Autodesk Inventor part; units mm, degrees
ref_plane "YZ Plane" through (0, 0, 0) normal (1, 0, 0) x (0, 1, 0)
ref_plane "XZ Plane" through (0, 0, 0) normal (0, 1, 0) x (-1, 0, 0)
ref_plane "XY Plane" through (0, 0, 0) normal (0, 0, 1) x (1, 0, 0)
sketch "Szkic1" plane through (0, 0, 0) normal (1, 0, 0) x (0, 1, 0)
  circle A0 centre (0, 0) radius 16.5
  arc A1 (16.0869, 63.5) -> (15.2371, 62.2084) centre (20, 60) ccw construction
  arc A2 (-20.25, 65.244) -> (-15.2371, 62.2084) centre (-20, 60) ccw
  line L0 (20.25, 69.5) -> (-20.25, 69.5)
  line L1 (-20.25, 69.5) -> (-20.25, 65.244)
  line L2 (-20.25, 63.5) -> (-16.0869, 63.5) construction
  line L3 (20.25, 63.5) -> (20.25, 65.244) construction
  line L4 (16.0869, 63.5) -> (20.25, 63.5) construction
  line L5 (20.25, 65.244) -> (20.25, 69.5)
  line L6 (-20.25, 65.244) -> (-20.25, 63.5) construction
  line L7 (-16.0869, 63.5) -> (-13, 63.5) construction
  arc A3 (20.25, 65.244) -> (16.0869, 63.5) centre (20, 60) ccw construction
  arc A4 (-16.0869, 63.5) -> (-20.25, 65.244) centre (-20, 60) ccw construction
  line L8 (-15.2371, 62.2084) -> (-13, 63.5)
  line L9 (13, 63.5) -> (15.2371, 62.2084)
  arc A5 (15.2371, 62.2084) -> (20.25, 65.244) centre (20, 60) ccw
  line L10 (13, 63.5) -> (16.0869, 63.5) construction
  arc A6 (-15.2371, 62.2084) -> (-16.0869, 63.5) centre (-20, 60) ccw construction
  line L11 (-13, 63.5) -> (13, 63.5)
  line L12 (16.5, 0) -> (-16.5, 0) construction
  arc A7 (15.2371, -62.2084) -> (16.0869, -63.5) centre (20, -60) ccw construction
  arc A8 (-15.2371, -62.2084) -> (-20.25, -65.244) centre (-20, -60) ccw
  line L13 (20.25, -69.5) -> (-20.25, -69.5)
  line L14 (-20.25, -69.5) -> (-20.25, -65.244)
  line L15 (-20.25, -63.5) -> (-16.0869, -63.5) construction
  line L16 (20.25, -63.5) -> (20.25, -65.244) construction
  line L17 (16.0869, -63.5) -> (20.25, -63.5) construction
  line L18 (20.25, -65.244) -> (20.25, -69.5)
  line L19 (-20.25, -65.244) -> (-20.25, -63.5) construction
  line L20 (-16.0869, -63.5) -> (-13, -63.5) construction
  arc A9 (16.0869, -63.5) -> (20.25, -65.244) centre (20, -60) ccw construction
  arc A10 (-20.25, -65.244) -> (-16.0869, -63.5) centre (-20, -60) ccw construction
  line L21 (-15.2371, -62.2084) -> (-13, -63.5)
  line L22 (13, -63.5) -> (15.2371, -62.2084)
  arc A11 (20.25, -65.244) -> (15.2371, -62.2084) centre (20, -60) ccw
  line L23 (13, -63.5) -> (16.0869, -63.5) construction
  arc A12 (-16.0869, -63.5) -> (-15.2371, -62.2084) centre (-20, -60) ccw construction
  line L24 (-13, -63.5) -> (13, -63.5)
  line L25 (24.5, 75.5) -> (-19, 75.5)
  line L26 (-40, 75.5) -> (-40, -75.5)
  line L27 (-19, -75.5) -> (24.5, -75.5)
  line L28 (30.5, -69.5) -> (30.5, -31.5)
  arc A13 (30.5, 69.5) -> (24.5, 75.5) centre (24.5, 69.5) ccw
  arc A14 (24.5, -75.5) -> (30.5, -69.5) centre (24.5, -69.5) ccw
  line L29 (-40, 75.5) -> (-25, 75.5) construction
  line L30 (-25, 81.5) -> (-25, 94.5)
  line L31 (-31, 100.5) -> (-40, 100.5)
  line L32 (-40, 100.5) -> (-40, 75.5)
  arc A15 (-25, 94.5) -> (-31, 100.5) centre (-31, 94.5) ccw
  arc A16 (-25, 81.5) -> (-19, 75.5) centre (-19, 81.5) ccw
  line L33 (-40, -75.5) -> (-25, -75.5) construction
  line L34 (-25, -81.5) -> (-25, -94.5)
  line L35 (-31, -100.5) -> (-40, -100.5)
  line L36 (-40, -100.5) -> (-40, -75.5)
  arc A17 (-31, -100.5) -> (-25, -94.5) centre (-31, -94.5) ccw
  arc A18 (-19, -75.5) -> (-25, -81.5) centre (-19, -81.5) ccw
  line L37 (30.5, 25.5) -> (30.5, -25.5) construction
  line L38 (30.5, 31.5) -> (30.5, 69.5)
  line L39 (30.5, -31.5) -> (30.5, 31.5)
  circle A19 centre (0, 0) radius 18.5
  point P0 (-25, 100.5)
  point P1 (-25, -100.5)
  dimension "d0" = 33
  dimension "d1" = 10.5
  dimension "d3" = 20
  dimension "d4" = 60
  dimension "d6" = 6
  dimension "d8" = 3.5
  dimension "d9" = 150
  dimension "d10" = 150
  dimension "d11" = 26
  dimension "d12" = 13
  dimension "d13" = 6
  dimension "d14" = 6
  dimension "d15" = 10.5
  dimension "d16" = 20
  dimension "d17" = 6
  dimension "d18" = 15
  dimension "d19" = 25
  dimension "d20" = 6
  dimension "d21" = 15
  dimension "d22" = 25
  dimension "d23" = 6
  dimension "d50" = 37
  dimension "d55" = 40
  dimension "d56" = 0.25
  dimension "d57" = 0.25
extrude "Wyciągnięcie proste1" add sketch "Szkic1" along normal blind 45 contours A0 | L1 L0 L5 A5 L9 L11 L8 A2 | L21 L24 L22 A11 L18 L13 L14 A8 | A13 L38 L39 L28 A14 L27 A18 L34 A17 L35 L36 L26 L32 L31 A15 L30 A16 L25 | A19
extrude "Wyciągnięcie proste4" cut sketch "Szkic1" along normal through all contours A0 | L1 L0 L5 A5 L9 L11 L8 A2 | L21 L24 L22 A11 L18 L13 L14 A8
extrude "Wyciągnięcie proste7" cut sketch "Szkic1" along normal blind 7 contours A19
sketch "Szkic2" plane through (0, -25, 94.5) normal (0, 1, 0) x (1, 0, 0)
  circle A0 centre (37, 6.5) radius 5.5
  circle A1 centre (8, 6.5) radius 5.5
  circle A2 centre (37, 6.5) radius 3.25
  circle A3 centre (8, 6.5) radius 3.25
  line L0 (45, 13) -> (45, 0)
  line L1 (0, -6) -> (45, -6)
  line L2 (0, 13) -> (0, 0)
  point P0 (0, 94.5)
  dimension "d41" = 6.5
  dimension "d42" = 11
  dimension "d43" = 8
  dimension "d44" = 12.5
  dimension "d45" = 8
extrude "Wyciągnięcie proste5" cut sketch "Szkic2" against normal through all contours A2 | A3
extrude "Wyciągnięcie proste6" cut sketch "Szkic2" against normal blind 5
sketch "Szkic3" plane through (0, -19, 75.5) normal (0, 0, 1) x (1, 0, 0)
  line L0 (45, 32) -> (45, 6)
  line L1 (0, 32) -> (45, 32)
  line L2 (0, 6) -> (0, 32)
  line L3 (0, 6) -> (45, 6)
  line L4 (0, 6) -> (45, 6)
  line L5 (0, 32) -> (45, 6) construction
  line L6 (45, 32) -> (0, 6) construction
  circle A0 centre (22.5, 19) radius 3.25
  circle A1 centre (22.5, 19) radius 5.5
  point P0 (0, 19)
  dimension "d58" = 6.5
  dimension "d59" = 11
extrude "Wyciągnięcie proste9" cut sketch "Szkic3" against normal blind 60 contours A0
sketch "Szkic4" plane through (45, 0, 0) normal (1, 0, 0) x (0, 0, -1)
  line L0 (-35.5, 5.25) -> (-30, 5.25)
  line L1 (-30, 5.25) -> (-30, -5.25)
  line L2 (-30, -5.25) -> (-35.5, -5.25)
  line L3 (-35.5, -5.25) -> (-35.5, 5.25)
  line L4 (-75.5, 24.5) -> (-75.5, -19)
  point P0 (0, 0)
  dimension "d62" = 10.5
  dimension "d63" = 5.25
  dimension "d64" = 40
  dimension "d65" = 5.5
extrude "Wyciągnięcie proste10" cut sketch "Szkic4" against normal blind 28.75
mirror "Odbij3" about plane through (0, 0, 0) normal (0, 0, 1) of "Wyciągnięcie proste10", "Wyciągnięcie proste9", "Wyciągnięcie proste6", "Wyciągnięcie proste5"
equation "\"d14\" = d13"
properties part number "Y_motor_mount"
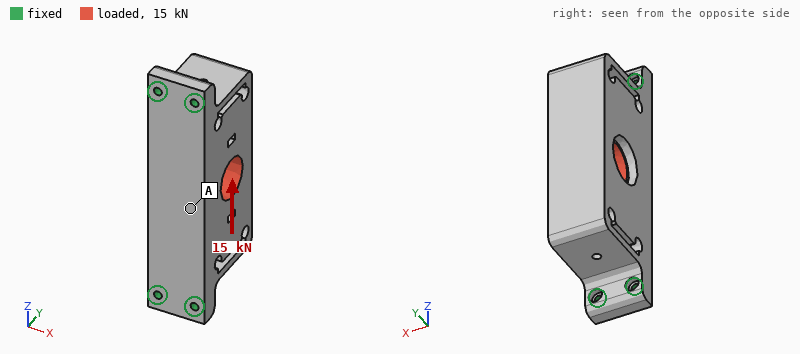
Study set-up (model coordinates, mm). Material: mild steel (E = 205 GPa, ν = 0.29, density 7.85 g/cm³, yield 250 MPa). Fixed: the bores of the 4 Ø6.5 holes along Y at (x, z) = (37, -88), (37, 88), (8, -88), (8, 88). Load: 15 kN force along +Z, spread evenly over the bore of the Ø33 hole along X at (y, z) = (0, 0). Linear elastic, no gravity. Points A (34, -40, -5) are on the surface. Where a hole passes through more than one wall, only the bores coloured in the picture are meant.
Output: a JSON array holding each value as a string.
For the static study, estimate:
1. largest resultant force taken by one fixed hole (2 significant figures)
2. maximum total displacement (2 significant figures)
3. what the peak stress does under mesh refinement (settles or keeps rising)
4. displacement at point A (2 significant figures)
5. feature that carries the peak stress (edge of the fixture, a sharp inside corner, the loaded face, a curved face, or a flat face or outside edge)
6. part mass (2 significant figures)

["4.3 kN", "10 µm", "keeps rising", "2.2 µm", "edge of the fixture", "3.3 kg"]
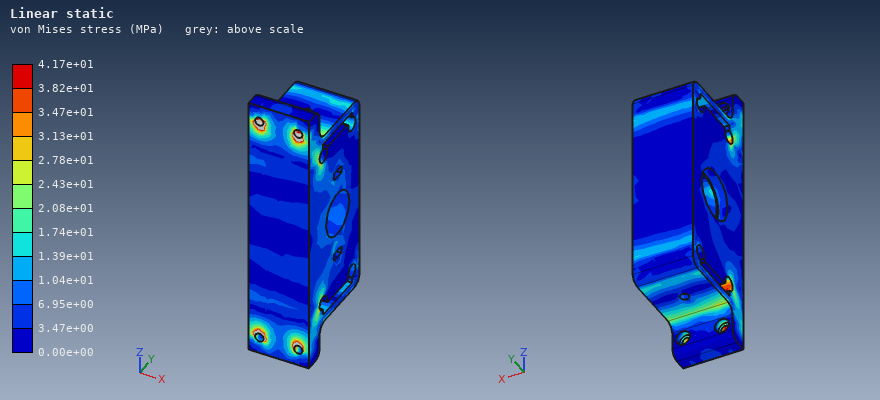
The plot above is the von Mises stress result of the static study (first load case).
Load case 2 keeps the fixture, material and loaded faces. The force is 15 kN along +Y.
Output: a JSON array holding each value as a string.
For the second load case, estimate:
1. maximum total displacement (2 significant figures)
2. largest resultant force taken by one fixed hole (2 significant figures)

["28 µm", "5.8 kN"]
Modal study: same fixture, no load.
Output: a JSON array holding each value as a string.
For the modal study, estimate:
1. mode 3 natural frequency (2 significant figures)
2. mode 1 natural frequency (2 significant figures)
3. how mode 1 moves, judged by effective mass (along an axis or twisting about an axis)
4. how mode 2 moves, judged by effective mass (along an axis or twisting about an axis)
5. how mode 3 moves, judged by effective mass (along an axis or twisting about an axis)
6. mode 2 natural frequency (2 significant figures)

["3700 Hz", "1700 Hz", "along X", "along Y", "along Z", "2500 Hz"]
